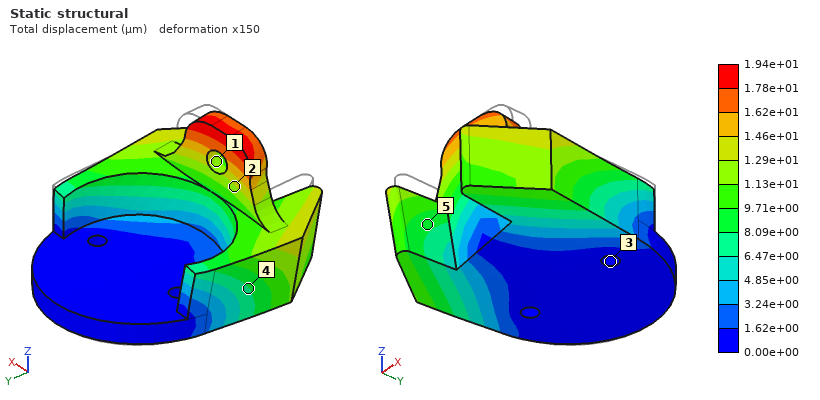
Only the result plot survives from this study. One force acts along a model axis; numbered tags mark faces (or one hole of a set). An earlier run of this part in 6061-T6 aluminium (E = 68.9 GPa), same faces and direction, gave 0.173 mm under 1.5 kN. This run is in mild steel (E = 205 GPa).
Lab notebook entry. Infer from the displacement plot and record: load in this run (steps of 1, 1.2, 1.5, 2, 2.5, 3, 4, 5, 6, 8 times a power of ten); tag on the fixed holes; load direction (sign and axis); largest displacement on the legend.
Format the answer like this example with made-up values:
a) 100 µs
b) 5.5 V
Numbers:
a) 500 N
b) 3
c) -X
d) 1.94e+01 µm
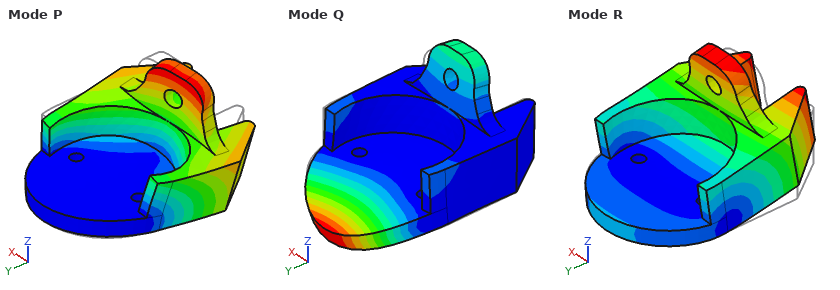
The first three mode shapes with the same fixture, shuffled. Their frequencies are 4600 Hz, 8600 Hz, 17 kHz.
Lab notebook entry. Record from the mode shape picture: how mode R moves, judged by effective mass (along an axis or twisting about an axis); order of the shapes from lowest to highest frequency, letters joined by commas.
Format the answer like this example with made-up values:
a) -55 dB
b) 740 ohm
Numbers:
a) along Z
b) R, P, Q
